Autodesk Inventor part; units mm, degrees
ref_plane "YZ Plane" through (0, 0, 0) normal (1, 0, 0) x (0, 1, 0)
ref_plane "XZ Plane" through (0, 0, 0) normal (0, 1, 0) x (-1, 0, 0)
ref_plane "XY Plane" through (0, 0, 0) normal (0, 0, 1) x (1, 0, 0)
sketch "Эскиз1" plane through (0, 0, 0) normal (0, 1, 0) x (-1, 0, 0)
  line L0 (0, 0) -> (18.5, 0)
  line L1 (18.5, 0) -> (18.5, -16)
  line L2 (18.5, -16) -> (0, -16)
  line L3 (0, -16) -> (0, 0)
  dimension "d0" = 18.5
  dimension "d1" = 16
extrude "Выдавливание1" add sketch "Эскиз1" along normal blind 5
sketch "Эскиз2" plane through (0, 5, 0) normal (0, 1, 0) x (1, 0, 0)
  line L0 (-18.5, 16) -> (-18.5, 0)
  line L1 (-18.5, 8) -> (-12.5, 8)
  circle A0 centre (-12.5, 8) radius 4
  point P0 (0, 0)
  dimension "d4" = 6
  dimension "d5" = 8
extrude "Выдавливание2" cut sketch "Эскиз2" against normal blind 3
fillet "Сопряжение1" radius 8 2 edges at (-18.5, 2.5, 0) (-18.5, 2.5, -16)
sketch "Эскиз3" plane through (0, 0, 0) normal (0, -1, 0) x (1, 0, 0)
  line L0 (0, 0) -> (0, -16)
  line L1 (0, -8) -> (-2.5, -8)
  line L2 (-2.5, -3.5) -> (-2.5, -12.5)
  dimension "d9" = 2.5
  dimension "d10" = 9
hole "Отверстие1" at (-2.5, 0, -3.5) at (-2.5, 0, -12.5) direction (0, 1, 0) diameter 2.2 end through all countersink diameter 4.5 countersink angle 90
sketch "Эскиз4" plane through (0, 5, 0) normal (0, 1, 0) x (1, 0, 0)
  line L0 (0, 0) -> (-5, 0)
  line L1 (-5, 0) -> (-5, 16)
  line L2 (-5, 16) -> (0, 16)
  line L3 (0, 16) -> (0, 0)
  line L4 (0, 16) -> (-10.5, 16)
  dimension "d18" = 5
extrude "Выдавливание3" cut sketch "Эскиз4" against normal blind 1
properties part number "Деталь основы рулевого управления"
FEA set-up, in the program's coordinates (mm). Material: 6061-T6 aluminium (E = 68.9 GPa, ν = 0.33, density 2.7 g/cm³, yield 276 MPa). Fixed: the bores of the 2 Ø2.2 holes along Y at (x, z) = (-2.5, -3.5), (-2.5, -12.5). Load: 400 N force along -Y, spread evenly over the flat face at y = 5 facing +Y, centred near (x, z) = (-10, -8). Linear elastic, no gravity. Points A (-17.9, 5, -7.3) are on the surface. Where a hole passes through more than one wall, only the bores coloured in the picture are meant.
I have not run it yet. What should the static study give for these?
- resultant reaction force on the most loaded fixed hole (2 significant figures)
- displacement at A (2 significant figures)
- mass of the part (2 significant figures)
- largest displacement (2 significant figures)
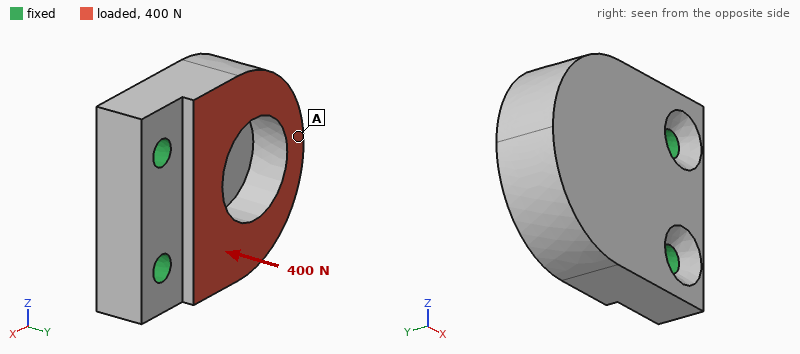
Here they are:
200 N
44 µm
2.9 g
46 µm
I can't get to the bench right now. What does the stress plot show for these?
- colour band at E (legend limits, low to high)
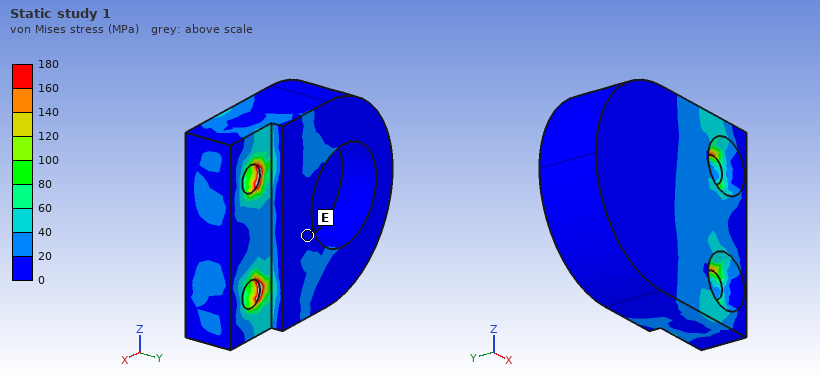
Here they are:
0 to 20 MPa
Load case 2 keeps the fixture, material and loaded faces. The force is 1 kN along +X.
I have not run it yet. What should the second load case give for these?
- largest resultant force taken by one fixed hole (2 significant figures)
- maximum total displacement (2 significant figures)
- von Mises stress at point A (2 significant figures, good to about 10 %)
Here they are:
500 N
52 µm
20 MPa
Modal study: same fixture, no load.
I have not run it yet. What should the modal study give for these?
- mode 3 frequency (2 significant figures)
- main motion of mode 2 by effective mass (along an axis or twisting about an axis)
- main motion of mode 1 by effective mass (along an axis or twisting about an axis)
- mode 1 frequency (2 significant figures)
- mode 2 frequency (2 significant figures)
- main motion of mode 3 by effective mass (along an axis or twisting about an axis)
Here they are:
34 kHz
along Z
along Y
13 kHz
29 kHz
along Z
